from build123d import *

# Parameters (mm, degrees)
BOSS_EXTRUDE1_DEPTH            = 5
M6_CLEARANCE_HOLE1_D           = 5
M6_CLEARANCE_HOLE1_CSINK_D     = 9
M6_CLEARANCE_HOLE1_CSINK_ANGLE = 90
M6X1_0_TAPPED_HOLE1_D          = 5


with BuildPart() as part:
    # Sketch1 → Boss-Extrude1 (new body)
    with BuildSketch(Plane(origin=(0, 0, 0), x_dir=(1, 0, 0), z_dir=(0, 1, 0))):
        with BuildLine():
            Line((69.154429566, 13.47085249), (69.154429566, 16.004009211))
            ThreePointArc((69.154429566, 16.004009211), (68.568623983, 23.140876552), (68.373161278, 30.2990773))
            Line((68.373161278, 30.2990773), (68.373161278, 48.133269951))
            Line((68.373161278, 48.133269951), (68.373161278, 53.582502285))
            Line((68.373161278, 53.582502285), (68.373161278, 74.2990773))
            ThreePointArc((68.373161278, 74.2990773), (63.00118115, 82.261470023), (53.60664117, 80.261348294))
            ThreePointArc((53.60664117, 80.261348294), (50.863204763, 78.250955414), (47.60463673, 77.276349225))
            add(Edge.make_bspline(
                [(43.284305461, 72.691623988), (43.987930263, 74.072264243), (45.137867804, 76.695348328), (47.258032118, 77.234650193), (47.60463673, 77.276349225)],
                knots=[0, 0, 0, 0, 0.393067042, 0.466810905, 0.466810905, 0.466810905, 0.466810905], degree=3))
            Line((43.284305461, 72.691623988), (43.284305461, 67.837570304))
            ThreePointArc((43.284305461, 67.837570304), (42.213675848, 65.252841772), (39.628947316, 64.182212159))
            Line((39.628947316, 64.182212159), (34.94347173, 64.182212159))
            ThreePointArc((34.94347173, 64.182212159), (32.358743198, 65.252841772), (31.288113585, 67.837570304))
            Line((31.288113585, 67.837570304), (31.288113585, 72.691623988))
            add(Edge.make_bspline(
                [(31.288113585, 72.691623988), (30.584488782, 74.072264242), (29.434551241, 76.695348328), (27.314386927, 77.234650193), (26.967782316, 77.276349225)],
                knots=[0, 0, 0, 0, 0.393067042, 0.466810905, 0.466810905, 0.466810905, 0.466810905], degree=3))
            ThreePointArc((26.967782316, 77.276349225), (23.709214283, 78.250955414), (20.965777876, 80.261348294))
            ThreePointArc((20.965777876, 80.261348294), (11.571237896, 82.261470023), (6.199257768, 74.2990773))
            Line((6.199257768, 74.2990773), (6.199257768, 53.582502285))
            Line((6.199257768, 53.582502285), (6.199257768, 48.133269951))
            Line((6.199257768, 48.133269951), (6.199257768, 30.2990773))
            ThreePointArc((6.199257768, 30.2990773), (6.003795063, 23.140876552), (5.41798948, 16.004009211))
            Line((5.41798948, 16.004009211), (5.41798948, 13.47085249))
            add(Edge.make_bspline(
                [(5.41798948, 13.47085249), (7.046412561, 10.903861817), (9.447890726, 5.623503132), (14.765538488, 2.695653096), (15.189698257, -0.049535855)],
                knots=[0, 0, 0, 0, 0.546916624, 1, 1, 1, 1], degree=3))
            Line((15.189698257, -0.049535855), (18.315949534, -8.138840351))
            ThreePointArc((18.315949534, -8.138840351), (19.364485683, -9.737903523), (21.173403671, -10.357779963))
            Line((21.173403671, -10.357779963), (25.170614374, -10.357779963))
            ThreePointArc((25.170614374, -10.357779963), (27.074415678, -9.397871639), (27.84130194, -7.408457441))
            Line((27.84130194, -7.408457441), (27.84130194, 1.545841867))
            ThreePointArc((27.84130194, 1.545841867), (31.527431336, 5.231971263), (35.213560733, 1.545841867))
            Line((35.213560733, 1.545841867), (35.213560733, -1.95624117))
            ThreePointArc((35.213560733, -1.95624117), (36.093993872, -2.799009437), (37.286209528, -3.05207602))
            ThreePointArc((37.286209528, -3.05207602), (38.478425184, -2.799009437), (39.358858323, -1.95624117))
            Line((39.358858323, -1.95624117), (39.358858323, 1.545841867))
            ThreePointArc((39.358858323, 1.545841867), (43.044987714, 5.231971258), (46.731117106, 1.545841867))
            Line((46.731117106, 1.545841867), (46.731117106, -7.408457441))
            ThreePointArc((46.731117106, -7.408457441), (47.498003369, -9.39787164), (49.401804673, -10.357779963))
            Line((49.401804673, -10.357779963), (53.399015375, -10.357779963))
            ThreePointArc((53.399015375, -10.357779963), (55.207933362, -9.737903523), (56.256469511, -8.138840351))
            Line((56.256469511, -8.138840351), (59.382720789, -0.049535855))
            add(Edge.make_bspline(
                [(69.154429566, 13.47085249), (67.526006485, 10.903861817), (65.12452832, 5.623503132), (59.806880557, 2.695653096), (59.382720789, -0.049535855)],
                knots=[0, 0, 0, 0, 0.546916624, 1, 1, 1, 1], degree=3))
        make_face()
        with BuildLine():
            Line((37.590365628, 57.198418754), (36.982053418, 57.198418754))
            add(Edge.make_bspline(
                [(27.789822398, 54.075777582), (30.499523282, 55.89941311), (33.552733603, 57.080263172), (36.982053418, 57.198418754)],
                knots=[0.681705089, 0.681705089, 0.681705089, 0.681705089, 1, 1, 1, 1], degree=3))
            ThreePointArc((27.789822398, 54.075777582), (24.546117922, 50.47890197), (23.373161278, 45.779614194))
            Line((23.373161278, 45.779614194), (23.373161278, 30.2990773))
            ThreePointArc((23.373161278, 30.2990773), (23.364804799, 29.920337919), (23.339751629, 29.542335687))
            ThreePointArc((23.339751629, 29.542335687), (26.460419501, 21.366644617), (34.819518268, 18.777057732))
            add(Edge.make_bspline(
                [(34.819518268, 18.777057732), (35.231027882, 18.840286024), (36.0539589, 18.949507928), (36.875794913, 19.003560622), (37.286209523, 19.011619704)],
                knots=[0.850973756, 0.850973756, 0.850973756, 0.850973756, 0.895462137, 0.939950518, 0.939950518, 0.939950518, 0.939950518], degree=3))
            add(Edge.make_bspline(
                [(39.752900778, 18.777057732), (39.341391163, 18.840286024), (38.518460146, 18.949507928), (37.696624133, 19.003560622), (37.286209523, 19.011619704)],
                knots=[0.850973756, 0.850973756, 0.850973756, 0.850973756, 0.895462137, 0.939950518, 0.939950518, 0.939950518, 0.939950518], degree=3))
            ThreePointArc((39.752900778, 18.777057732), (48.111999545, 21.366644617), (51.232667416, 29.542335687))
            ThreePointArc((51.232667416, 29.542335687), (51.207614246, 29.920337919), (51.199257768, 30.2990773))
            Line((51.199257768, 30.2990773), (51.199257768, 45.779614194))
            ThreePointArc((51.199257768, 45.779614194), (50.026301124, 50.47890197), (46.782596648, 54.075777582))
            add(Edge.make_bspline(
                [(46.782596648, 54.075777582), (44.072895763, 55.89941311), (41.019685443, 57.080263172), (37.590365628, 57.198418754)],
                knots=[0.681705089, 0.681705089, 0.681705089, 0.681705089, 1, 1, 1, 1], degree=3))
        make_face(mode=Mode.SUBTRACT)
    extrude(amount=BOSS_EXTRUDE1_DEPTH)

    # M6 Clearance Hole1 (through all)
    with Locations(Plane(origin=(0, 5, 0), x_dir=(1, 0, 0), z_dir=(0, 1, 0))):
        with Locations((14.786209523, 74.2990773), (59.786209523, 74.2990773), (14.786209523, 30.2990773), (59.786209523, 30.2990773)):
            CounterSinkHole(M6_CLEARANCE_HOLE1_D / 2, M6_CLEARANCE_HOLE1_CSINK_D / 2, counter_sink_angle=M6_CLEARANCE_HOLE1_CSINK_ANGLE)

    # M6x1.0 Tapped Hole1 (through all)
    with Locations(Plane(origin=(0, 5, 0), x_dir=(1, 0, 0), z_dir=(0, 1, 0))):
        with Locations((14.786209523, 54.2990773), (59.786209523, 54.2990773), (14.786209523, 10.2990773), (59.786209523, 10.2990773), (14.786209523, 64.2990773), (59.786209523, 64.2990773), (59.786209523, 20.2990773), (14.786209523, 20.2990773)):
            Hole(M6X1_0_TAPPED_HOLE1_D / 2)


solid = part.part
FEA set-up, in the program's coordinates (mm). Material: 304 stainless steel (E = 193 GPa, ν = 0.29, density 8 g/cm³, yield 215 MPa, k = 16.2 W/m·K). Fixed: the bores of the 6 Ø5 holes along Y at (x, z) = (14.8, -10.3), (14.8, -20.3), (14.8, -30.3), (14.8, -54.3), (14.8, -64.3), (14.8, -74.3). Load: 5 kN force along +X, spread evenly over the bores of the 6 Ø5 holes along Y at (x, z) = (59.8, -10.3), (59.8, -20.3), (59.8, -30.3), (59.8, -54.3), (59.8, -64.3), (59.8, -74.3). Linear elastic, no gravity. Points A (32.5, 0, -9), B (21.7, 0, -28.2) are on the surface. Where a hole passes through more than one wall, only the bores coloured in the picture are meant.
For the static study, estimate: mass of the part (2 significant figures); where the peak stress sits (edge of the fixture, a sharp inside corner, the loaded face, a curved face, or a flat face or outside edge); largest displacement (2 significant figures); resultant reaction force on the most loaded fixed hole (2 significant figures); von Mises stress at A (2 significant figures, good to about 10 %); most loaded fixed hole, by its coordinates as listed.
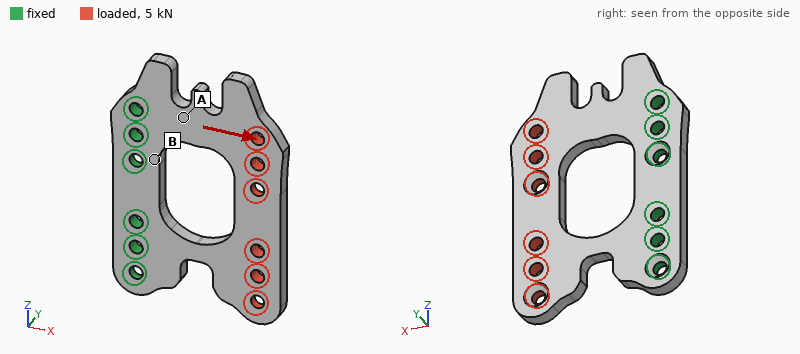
140 g
a curved face
34 µm
1.6 kN
33 MPa
(14.8, -10.3)
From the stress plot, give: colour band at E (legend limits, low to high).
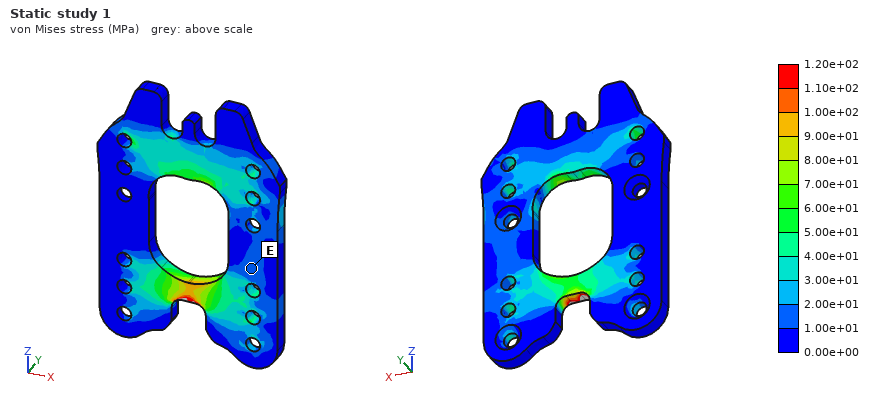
1.00e+01 to 2.00e+01 MPa
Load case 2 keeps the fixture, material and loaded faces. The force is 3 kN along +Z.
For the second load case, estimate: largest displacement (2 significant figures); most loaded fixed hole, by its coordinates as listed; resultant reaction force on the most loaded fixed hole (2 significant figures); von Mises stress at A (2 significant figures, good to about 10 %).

50 µm
(14.8, -10.3)
3.3 kN
65 MPa
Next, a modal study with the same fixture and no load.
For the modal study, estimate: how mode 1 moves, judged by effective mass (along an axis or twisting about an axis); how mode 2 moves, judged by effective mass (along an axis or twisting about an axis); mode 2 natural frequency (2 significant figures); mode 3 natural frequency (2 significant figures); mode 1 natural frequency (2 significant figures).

along Y
twisting about X
1800 Hz
3900 Hz
1000 Hz
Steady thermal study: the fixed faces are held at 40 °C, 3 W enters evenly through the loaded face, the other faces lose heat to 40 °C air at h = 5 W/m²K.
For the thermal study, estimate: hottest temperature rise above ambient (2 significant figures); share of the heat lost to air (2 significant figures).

43 K
30 %
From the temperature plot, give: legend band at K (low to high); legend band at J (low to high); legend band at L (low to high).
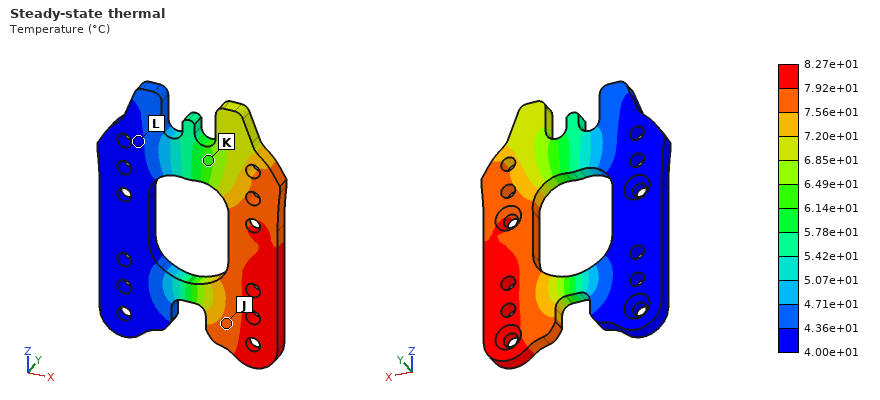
6.14e+01 to 6.49e+01 °C
7.56e+01 to 7.92e+01 °C
4.00e+01 to 4.36e+01 °C
